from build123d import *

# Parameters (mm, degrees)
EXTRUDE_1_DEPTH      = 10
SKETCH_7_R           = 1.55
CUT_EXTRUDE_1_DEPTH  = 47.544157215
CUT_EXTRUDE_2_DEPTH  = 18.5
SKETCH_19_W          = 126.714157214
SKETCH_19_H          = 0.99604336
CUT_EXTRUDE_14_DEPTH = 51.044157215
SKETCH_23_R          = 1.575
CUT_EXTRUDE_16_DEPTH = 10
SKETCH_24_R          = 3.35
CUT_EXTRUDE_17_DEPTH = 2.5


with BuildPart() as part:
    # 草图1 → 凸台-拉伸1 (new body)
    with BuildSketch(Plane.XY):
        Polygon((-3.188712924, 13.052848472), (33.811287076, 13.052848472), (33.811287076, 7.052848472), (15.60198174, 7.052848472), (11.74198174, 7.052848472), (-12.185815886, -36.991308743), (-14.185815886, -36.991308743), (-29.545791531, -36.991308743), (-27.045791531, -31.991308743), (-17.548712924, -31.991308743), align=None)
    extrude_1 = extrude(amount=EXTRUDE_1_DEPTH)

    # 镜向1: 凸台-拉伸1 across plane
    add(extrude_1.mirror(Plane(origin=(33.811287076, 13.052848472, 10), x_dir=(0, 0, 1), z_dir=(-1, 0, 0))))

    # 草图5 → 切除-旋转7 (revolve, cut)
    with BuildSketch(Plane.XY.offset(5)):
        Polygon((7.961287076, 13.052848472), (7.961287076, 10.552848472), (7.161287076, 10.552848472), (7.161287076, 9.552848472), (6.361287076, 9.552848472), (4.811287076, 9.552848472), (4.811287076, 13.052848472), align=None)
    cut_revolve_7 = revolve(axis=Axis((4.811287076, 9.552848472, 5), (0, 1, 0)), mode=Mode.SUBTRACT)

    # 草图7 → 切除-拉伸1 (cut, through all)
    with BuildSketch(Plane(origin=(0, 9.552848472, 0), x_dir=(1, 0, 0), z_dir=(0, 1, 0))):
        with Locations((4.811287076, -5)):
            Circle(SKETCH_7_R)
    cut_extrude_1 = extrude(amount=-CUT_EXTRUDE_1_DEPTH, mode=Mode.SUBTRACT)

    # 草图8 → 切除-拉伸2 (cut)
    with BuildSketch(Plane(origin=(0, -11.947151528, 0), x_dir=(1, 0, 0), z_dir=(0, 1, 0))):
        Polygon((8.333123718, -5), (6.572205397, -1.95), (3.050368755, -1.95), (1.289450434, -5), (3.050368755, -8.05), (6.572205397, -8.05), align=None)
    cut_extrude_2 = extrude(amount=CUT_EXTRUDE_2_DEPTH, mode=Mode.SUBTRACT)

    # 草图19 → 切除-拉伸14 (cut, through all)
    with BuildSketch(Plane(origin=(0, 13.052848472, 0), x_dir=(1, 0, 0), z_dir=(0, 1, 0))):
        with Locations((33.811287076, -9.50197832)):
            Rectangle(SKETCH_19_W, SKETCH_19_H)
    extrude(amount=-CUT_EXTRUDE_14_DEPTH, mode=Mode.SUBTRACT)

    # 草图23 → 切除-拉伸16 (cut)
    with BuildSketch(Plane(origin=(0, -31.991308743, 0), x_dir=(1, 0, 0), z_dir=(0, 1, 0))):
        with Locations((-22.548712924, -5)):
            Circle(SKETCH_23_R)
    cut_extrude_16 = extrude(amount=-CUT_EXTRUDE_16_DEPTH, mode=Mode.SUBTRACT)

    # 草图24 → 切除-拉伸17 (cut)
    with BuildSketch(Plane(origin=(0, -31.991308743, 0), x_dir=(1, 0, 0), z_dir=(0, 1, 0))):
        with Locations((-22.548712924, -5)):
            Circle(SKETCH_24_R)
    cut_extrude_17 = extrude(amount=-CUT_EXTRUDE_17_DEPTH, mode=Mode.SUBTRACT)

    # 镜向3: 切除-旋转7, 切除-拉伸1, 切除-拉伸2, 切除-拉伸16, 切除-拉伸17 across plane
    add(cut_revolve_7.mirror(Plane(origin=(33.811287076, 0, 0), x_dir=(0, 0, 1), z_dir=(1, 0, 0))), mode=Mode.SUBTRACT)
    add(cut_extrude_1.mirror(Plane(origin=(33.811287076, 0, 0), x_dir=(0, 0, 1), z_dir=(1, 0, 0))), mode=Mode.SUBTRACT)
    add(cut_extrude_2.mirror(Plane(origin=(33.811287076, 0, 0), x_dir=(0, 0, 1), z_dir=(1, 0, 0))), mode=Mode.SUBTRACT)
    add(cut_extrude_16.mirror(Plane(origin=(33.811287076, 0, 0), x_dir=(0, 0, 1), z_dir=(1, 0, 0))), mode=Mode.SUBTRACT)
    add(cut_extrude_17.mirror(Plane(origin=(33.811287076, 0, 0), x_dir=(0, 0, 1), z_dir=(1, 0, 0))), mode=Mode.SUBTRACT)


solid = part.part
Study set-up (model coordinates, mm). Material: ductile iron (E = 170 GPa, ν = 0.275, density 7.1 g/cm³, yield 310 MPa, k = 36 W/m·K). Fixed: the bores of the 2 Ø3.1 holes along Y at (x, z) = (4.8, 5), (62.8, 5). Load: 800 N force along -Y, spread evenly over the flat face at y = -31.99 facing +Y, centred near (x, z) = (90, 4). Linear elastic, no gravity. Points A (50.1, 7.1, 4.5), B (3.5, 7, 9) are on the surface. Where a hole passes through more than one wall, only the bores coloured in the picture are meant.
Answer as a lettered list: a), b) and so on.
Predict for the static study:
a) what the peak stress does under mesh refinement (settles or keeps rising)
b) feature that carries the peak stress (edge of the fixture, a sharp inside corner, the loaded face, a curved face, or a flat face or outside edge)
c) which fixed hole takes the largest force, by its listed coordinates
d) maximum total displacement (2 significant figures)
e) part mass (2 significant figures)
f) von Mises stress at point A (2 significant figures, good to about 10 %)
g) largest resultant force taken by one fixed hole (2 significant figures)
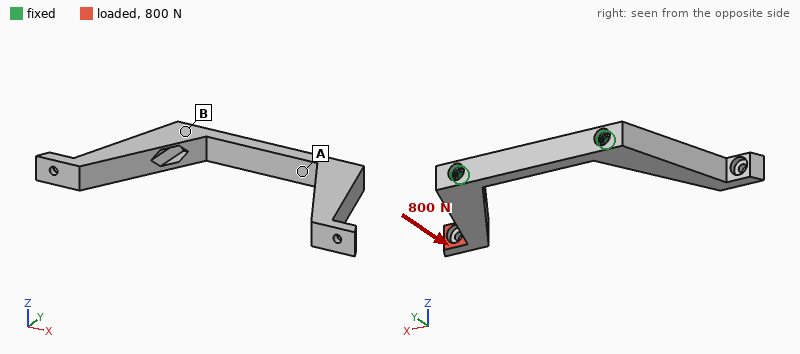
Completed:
a) keeps rising
b) edge of the fixture
c) (62.8, 5)
d) 0.32 mm
e) 94 g
f) 60 MPa
g) 1.2 kN
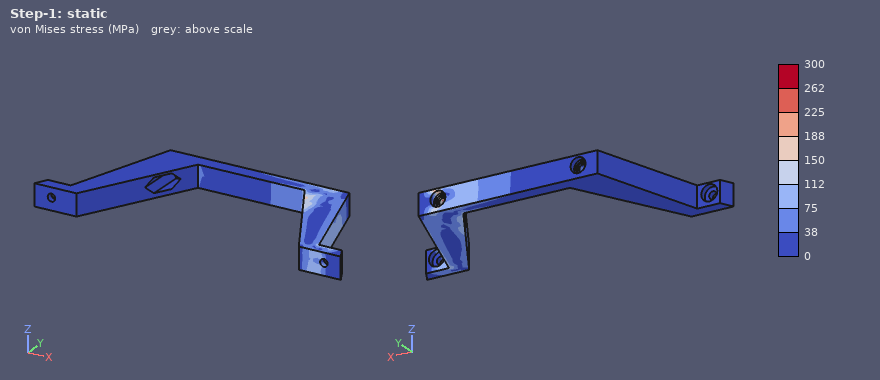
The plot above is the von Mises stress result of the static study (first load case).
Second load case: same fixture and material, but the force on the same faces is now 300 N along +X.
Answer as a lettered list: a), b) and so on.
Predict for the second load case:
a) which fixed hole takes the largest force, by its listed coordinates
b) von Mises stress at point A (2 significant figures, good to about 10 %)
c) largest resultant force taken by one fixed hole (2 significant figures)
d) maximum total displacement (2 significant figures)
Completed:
a) (62.8, 5)
b) 35 MPa
c) 680 N
d) 0.15 mm
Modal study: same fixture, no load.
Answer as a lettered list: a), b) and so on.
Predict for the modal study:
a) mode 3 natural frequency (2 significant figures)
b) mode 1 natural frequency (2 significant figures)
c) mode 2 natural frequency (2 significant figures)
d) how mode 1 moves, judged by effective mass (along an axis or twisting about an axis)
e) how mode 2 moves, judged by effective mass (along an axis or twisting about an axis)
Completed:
a) 2000 Hz
b) 1800 Hz
c) 1900 Hz
d) along Z
e) twisting about Y
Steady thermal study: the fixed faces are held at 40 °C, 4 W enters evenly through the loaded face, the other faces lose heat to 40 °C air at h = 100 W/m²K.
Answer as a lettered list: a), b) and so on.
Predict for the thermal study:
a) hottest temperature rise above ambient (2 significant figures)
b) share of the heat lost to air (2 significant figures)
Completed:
a) 40 K
b) 80 %
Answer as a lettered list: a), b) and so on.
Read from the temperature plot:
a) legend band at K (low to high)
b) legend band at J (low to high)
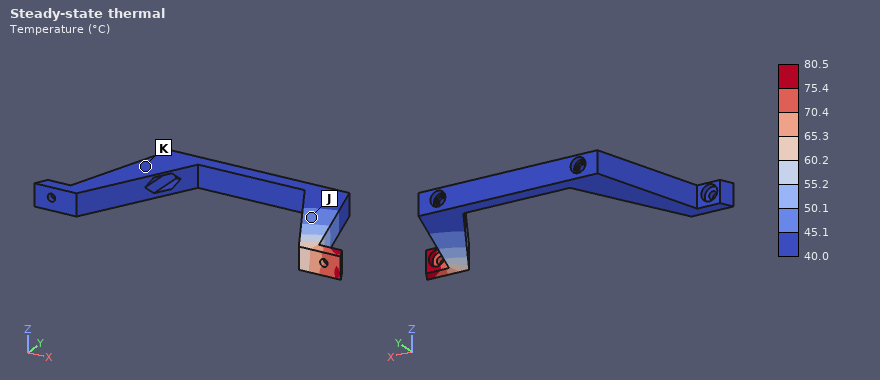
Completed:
a) 40.0 to 45.1 °C
b) 45.1 to 50.1 °C
